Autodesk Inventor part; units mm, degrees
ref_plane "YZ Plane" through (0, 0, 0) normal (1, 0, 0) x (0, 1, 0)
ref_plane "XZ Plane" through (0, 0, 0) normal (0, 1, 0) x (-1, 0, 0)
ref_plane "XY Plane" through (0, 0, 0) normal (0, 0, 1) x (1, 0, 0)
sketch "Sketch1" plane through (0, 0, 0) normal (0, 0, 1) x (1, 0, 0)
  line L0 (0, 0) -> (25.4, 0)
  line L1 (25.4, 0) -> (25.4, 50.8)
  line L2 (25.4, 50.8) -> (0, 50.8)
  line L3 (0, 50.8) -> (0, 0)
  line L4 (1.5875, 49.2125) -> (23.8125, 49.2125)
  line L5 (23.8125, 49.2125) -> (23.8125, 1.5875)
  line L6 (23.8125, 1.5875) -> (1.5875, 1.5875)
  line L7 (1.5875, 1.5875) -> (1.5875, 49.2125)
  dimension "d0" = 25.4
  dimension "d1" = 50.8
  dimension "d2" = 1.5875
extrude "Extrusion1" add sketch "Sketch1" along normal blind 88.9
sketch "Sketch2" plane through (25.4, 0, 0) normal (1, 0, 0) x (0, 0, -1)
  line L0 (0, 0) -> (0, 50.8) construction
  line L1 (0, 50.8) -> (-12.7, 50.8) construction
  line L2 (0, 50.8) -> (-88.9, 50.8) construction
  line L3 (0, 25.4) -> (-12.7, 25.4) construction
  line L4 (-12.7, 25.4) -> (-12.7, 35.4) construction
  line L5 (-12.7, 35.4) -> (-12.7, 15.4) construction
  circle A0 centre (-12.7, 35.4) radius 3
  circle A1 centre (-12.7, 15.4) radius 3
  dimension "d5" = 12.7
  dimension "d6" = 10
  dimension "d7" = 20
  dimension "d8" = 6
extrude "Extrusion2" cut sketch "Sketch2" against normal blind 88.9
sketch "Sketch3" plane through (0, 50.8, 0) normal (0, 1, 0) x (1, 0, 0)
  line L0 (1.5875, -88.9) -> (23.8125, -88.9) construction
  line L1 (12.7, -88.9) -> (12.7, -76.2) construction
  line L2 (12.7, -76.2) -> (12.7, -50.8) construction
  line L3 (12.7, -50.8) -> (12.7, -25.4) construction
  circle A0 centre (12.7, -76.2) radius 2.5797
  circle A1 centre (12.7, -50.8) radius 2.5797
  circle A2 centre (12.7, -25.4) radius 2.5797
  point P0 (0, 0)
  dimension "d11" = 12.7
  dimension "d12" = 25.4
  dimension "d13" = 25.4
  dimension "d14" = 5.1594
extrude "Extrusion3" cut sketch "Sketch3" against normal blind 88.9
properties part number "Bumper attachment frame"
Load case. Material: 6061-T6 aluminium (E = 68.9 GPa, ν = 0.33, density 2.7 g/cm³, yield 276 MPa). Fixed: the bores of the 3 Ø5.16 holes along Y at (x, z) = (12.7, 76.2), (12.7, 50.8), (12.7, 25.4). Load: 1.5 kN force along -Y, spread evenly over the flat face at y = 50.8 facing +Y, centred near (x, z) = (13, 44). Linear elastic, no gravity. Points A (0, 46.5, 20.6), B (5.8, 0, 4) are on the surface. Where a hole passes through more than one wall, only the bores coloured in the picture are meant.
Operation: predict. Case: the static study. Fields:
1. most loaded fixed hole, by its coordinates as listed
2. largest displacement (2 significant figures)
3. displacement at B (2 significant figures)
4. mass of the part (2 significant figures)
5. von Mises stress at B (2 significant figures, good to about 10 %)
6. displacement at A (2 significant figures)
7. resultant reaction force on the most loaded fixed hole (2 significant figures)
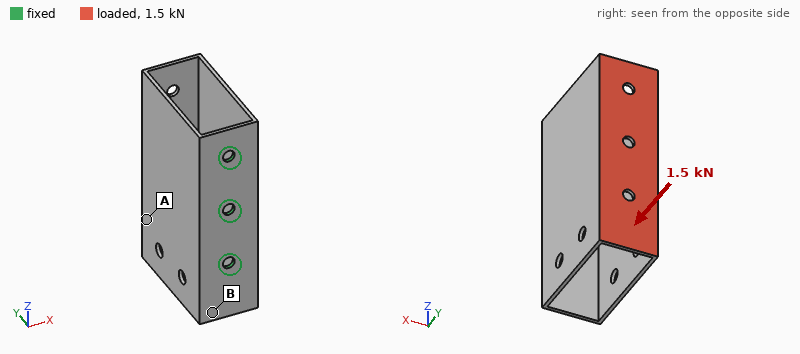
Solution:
(12.7, 25.4)
0.29 mm
0.13 mm
55 g
40 MPa
0.16 mm
690 N
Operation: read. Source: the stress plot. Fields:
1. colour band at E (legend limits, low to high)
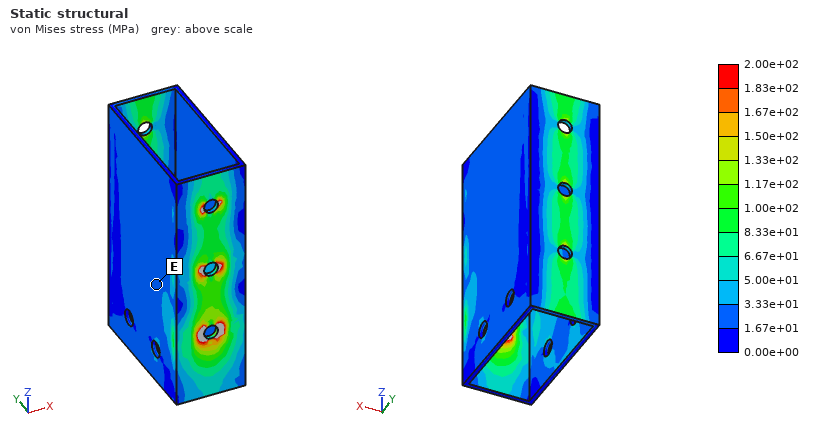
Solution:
1.67e+01 to 3.33e+01 MPa
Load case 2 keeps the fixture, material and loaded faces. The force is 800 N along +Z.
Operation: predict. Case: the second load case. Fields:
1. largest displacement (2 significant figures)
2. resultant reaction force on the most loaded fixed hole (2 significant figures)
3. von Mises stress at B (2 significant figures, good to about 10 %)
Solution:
0.42 mm
780 N
36 MPa
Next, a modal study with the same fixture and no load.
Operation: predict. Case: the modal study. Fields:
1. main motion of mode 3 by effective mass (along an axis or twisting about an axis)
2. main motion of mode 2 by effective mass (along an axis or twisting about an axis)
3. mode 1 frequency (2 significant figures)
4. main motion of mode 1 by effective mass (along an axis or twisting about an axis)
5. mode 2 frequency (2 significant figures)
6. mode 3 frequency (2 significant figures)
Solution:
along Z
twisting about Y
420 Hz
along X
1300 Hz
1400 Hz
